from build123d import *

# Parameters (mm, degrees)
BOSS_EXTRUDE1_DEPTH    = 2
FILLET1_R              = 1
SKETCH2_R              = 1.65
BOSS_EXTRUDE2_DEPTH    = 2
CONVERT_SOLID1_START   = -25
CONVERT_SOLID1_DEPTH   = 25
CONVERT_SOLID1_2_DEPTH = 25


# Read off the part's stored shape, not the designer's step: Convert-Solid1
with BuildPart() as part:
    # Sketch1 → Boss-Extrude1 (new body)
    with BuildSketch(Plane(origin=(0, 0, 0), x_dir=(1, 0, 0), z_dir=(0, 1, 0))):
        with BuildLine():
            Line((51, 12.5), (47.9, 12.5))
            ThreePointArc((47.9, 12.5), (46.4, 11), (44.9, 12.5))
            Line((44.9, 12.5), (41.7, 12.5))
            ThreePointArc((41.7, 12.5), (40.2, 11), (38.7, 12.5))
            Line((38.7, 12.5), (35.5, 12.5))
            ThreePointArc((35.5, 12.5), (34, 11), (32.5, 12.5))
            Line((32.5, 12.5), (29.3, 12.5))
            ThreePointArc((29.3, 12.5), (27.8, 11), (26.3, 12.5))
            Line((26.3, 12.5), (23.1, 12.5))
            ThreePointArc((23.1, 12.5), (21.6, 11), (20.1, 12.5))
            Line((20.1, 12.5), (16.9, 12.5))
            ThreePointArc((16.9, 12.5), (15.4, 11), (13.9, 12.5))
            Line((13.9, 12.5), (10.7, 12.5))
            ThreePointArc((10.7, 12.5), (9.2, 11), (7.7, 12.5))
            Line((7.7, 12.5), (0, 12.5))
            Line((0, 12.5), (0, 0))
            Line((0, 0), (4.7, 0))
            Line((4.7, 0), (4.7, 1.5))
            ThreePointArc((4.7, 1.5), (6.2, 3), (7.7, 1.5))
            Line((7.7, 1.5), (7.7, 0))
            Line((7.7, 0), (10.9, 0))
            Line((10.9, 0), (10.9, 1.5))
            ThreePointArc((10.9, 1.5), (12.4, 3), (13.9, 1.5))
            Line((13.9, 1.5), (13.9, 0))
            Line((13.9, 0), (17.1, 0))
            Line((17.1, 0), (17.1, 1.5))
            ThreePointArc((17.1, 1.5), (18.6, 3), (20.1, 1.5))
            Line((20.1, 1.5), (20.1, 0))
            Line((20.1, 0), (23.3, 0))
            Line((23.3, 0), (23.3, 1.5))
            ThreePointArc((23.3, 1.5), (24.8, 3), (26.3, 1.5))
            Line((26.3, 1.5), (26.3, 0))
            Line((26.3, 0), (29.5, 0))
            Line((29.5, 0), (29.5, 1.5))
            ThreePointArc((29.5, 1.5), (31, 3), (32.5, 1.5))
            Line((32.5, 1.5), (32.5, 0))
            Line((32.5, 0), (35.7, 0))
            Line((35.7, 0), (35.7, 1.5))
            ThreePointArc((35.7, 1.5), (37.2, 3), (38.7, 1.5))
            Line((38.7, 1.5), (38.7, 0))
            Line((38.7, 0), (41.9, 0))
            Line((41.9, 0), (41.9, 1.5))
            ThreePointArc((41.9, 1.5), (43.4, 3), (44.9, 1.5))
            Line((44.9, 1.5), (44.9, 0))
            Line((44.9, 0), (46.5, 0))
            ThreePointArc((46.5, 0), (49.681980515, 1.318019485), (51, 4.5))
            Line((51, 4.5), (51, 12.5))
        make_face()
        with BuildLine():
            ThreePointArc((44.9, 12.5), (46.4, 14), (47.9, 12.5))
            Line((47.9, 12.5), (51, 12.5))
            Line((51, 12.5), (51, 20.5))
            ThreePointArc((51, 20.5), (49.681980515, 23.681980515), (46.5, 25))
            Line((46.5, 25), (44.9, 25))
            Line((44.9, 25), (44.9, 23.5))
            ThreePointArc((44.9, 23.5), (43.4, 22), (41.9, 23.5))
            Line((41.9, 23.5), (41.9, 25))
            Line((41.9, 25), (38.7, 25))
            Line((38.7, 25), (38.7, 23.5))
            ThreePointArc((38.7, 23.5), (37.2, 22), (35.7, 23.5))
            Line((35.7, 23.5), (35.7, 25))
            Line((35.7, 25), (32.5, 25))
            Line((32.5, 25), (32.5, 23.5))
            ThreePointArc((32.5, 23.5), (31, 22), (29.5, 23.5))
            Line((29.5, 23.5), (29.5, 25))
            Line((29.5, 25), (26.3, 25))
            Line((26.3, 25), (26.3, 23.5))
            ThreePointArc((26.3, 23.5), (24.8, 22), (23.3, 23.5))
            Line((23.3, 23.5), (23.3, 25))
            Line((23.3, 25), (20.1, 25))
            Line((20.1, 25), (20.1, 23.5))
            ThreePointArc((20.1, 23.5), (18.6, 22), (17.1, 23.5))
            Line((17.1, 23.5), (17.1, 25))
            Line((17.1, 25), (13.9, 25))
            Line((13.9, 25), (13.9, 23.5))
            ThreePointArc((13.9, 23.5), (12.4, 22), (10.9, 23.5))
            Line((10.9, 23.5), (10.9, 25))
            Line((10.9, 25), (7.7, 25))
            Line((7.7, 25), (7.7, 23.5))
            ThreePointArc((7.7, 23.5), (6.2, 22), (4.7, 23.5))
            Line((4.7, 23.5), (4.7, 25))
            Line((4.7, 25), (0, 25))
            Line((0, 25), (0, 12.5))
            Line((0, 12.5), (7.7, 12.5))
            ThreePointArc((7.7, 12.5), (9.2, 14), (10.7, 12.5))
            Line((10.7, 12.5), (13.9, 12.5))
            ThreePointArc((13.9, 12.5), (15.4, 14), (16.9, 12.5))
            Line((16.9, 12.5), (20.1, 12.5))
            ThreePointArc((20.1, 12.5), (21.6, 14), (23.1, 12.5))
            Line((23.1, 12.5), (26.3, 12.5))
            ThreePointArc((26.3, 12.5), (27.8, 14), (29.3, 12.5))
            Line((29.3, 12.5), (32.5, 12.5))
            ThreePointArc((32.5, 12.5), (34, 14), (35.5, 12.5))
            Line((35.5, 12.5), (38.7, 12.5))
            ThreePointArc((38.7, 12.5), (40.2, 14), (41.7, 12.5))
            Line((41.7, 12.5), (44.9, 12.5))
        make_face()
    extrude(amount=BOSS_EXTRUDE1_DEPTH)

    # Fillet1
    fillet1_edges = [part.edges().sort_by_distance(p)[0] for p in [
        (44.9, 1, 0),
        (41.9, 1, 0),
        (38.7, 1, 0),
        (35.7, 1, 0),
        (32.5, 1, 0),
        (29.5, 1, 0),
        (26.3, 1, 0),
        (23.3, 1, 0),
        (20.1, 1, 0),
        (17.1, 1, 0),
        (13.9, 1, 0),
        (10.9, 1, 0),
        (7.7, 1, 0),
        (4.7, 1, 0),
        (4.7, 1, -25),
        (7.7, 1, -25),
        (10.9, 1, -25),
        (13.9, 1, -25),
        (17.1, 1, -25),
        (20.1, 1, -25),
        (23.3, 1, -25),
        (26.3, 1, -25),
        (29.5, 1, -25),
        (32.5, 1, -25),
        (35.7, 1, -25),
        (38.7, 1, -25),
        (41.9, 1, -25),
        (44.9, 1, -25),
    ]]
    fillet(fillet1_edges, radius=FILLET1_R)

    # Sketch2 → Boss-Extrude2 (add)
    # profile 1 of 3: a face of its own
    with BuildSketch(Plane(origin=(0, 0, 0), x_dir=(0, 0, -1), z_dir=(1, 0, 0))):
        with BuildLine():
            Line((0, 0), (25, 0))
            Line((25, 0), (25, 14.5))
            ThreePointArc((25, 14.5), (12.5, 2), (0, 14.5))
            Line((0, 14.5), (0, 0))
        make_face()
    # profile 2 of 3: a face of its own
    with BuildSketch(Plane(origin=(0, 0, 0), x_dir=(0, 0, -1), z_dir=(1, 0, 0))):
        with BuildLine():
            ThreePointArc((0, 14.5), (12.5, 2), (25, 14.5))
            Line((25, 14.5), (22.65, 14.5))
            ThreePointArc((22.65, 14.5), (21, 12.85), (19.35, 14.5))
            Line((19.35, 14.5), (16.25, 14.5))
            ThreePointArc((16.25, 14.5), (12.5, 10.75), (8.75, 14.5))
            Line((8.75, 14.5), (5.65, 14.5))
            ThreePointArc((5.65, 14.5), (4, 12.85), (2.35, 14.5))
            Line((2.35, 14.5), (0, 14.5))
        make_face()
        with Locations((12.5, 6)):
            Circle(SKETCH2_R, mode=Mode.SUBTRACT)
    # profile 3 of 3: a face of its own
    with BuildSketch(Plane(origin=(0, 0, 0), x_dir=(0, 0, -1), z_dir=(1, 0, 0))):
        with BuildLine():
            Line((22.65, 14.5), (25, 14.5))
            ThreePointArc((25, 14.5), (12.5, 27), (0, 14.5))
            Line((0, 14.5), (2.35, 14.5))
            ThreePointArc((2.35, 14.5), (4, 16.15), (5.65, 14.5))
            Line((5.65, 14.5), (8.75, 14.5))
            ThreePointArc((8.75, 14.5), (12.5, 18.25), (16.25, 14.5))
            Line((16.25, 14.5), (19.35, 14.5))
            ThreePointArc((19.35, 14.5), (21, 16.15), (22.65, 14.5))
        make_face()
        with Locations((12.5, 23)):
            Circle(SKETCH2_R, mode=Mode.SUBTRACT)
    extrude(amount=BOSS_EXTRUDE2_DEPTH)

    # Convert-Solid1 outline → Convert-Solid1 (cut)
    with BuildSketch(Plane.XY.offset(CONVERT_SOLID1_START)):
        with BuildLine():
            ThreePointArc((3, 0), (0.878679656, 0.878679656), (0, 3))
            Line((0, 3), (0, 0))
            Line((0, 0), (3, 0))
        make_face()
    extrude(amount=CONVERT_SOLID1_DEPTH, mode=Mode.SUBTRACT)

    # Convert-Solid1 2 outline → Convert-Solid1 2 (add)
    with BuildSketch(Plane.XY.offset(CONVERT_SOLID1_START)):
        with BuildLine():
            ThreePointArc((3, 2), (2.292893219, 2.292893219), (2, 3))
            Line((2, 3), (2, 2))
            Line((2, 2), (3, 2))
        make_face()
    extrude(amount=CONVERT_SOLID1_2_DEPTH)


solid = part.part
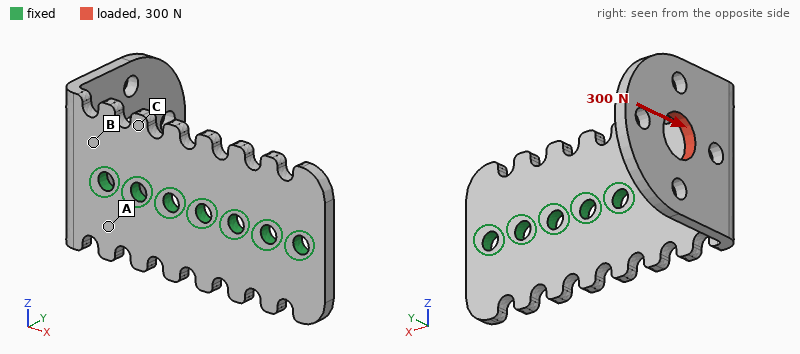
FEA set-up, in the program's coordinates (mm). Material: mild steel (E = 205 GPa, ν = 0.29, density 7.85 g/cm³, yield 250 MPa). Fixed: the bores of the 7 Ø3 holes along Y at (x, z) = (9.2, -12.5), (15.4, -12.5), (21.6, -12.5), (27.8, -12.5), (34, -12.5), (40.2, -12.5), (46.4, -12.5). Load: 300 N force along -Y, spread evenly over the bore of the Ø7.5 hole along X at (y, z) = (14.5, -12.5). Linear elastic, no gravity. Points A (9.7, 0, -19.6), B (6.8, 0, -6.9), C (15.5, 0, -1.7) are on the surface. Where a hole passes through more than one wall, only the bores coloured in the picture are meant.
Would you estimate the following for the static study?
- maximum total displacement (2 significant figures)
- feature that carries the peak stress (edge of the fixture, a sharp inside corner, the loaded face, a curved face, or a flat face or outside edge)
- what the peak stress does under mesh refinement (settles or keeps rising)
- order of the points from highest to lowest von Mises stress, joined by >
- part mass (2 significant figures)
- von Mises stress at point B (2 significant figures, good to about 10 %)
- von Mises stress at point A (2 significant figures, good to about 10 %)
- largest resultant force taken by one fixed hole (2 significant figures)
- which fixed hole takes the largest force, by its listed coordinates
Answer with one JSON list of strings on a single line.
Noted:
["98 µm", "edge of the fixture", "keeps rising", "B > A > C", "24 g", "89 MPa", "62 MPa", "410 N", "(9.2, -12.5)"]
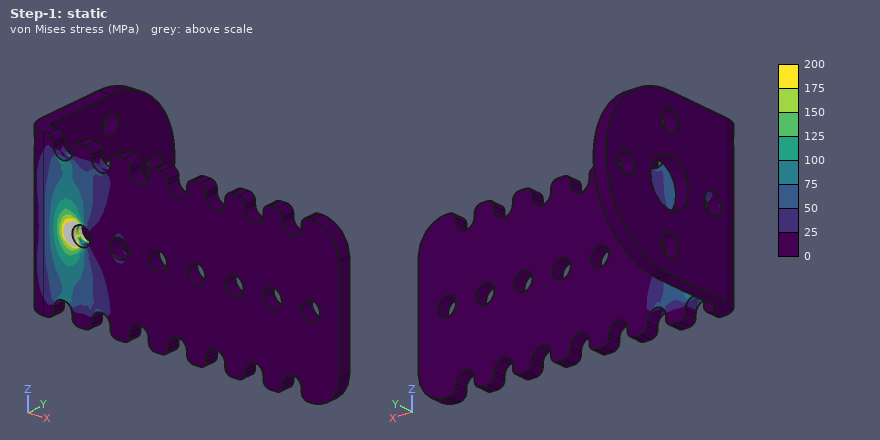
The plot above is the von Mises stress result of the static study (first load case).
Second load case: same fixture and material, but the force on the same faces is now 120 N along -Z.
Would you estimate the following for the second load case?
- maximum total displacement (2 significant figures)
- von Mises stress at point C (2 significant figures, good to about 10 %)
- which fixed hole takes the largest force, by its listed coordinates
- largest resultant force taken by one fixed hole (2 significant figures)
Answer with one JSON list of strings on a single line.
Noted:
["67 µm", "7.9 MPa", "(9.2, -12.5)", "160 N"]
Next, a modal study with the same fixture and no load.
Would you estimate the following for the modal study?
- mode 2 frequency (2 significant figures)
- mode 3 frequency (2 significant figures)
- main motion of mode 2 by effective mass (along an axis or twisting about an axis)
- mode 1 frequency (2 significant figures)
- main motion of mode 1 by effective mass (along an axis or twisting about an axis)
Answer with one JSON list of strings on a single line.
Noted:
["2900 Hz", "6700 Hz", "along Z", "1900 Hz", "along X"]
